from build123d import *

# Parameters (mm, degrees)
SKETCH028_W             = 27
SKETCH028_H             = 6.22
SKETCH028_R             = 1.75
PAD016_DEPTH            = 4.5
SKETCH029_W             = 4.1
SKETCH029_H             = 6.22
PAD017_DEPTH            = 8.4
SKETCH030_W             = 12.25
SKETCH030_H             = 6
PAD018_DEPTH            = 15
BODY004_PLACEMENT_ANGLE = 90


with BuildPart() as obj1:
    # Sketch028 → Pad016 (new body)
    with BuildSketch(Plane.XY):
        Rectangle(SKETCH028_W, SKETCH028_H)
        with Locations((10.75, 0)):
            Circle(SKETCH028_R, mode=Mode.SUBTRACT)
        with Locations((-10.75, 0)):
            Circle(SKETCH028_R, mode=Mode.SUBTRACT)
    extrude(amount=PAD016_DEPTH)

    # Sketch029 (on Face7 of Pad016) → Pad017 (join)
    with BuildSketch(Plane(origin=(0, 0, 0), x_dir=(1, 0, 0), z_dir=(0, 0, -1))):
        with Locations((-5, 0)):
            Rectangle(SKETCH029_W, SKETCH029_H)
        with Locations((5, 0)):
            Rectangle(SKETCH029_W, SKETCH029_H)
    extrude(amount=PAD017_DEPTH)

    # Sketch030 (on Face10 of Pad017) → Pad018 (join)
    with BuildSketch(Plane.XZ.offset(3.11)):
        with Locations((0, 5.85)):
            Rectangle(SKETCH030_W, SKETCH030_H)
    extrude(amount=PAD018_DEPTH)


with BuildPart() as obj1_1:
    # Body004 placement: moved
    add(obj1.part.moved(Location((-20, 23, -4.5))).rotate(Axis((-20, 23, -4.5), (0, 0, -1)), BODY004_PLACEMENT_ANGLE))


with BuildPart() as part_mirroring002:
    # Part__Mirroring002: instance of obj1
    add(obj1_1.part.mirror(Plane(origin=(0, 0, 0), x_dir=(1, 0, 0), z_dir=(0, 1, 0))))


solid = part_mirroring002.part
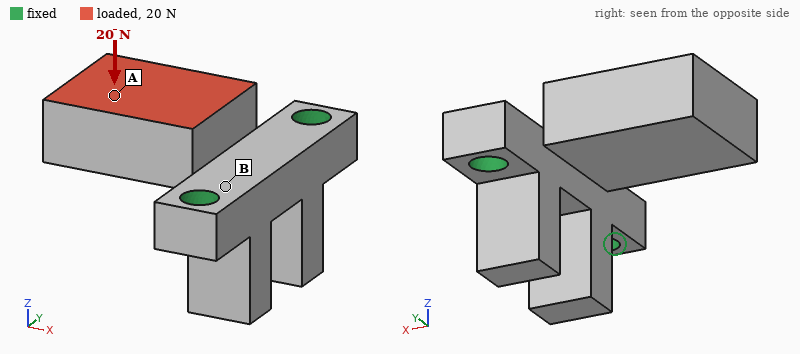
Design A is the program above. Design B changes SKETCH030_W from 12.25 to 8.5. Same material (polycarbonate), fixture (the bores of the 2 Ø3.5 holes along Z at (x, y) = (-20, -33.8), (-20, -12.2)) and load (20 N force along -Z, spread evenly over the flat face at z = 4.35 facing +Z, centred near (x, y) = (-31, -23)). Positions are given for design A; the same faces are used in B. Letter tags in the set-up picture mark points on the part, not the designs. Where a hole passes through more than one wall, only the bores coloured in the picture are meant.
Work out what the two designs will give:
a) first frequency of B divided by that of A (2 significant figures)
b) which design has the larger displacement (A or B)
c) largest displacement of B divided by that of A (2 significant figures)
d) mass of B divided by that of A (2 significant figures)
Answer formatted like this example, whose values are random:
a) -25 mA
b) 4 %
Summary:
a) 1.0
b) B
c) 1.4
d) 0.85
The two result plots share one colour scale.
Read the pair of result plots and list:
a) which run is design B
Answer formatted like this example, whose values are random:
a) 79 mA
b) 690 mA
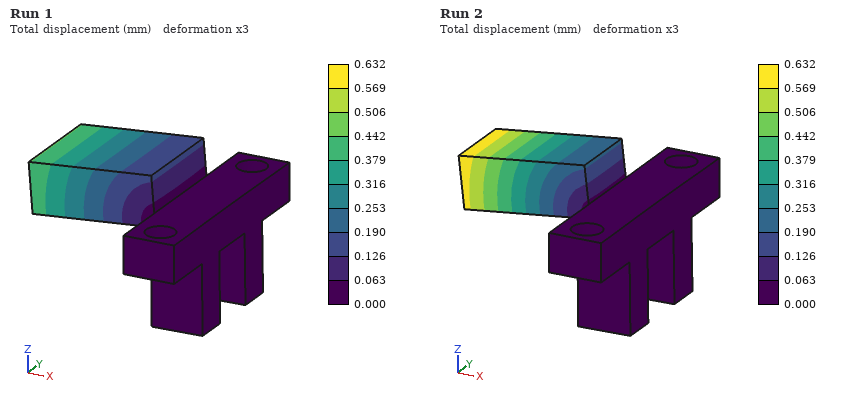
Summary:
a) Run 2
